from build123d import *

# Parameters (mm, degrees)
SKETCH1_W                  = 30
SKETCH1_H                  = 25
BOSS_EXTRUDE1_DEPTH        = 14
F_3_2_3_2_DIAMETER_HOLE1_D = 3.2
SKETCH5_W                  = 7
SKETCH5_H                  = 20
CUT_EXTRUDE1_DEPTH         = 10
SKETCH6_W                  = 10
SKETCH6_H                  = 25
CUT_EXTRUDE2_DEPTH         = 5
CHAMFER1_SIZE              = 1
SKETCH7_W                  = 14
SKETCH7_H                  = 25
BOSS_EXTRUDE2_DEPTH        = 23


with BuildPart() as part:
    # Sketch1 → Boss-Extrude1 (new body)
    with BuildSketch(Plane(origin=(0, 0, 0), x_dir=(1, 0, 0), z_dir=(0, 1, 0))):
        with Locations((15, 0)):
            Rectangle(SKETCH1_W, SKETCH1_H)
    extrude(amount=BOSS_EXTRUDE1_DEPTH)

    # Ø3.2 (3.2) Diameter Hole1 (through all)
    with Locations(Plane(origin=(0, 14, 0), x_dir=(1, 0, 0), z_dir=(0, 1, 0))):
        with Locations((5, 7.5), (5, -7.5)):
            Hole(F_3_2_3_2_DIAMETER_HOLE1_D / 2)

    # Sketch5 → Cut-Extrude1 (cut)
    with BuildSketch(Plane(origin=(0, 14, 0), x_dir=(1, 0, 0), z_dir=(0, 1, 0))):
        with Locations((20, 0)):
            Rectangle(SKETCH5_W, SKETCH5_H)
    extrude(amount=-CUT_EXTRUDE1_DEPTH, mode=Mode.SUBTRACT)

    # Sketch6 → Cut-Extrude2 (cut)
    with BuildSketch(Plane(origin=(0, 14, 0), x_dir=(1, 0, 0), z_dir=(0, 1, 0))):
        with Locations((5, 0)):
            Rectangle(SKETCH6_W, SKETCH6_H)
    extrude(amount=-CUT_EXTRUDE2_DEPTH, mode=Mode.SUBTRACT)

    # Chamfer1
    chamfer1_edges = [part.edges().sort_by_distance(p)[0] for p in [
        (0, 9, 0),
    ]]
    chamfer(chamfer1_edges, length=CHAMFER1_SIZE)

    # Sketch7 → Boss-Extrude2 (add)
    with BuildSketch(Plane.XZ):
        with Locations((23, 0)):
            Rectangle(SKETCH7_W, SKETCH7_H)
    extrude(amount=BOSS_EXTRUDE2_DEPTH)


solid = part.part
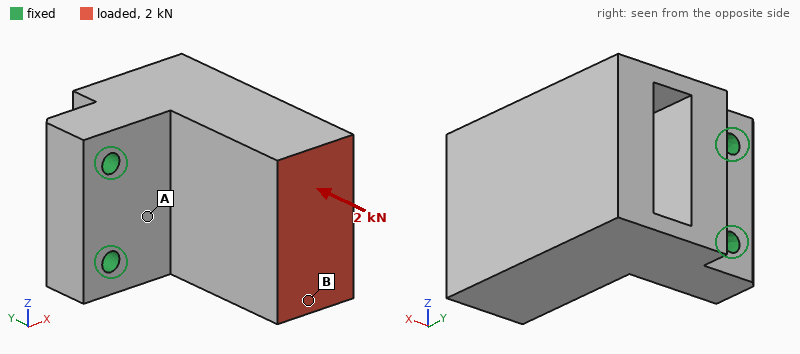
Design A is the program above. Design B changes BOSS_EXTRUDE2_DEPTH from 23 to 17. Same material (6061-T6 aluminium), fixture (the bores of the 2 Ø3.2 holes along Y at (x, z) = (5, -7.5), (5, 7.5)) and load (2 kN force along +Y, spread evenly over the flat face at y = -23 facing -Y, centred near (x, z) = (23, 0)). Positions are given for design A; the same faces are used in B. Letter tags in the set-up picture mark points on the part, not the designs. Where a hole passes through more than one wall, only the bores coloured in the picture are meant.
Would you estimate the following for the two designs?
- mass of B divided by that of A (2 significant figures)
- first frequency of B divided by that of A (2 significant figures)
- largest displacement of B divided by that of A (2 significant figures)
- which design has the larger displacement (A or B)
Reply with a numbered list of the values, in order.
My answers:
1. 0.87
2. 1.3
3. 0.87
4. A
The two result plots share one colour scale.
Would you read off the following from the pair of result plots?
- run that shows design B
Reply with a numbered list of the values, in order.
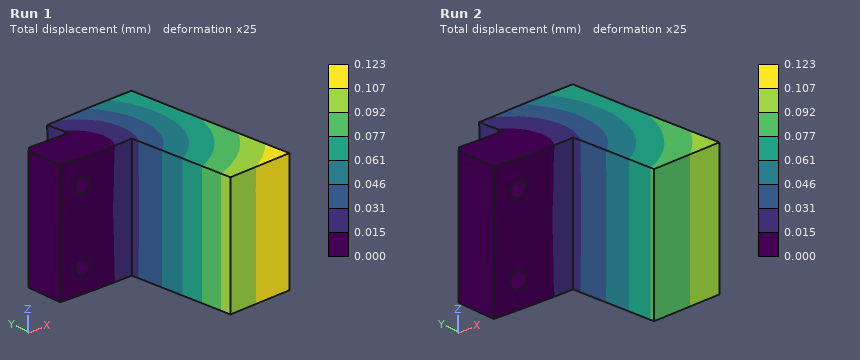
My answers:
1. Run 2
